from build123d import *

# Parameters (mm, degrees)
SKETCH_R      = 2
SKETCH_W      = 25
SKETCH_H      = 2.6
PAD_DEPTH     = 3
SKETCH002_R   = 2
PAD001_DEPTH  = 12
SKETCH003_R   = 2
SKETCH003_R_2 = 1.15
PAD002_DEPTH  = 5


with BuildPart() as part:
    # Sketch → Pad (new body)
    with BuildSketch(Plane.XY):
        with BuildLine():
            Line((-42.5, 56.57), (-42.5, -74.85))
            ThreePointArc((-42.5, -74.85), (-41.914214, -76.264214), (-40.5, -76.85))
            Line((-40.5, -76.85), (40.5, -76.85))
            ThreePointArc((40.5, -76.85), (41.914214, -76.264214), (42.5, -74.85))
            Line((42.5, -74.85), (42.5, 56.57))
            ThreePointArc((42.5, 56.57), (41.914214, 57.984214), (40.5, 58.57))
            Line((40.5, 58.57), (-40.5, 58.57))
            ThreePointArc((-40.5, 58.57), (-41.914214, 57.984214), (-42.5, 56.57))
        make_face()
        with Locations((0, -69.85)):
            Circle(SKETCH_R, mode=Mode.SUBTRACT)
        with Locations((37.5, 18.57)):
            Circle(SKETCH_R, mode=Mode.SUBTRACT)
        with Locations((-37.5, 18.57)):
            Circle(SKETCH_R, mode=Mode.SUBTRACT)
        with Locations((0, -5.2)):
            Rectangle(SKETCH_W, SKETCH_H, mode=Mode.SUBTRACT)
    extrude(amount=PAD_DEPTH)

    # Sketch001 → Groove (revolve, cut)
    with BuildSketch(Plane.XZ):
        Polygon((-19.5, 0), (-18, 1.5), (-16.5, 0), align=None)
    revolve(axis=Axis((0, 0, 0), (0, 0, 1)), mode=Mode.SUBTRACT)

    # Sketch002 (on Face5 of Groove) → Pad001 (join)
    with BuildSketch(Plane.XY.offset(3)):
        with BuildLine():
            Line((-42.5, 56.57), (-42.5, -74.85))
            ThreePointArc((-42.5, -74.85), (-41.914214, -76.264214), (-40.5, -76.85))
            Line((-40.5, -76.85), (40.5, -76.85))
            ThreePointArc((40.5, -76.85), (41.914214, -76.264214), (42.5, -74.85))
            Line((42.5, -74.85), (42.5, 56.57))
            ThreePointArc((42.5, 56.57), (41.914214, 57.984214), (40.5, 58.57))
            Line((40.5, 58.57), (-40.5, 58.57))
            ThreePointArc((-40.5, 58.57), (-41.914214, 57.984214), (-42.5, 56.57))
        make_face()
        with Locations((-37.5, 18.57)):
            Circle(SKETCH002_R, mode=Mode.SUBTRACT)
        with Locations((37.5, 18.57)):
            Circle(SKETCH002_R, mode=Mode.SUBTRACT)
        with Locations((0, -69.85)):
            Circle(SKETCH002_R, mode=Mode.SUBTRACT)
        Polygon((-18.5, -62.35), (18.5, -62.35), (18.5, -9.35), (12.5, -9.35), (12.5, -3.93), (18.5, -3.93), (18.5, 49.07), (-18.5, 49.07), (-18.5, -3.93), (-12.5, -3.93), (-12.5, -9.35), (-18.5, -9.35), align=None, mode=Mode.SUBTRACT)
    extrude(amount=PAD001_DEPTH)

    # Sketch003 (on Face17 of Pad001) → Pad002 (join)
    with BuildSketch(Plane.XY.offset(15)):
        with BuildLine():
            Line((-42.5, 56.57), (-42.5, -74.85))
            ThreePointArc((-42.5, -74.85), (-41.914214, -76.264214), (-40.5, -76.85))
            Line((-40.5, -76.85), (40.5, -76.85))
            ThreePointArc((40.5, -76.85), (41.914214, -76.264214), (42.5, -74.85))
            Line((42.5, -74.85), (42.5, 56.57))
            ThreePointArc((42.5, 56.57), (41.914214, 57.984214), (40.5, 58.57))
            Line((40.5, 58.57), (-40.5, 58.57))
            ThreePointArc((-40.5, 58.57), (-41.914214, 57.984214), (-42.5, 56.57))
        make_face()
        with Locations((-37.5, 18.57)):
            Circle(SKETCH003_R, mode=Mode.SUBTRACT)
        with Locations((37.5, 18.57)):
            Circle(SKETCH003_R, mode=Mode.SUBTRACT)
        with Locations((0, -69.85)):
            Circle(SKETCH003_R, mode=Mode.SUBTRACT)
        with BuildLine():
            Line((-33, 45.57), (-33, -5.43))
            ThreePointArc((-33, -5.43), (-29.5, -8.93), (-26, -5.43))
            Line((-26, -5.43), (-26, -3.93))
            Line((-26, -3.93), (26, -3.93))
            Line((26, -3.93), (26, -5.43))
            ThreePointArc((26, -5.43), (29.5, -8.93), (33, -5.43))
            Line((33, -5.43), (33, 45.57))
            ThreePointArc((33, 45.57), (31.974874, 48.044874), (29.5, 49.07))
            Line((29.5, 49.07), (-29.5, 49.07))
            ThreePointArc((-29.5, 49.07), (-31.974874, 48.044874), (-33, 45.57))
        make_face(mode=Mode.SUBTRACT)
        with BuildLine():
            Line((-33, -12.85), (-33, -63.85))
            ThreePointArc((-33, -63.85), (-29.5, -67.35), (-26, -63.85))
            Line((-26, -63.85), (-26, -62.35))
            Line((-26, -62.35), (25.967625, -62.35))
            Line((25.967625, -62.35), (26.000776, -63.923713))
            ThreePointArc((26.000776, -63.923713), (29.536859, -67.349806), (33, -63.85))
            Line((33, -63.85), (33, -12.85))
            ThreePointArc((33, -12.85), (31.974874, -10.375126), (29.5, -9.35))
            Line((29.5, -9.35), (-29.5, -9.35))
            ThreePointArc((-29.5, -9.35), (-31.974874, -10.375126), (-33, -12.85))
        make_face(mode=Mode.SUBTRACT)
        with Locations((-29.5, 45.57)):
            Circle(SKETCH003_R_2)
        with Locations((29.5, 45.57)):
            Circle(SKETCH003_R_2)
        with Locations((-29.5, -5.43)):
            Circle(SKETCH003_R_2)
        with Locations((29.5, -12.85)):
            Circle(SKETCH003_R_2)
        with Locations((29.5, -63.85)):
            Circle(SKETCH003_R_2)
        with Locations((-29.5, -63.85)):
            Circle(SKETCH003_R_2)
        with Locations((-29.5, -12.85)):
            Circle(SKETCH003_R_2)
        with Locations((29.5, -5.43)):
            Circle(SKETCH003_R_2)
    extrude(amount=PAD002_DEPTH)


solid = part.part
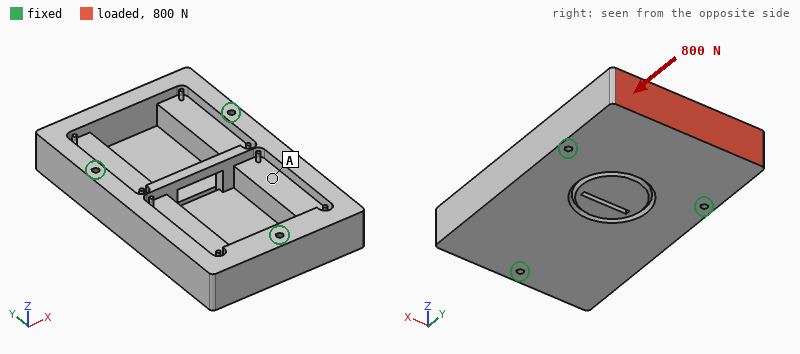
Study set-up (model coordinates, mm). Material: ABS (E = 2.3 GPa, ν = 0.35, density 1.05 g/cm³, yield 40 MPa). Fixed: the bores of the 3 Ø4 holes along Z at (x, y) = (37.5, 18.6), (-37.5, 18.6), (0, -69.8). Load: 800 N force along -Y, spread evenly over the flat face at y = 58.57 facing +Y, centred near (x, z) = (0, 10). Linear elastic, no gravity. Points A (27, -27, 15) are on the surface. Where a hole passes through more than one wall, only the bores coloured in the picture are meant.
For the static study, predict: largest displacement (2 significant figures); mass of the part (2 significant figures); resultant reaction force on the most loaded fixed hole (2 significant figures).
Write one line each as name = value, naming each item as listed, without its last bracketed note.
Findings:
largest displacement = 0.11 mm
mass of the part = 150 g
resultant reaction force on the most loaded fixed hole = 400 N
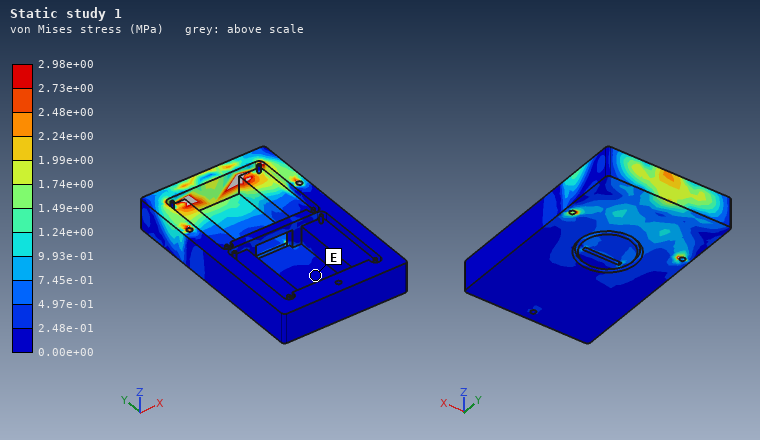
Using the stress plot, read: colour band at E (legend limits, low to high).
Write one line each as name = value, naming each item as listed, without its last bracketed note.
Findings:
colour band at E = 0.00e+00 to 2.48e-01 MPa
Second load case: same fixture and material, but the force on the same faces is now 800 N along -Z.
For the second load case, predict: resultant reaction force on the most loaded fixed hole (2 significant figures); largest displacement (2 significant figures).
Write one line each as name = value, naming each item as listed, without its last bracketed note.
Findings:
resultant reaction force on the most loaded fixed hole = 440 N
largest displacement = 0.60 mm
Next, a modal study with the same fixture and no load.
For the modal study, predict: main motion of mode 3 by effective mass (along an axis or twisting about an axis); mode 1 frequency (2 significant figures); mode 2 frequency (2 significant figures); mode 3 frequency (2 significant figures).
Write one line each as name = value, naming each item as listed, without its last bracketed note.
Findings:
main motion of mode 3 by effective mass = along Z
mode 1 frequency = 1500 Hz
mode 2 frequency = 1500 Hz
mode 3 frequency = 1700 Hz
